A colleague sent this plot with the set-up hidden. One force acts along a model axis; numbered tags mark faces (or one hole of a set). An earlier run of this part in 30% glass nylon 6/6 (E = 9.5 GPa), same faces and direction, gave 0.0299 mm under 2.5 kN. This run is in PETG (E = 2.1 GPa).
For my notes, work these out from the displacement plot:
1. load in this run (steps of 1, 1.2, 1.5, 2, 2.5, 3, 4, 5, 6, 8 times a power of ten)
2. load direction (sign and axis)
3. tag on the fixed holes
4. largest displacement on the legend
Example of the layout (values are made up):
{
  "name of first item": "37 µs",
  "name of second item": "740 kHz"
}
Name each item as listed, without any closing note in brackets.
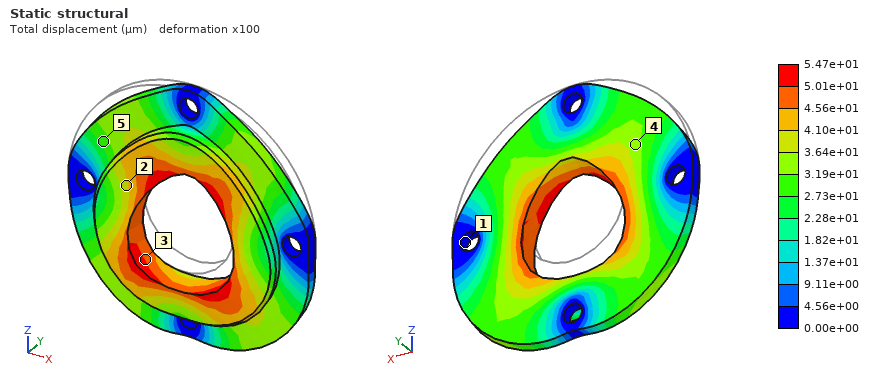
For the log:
{
  "load in this run": "1 kN",
  "load direction": "-Z",
  "tag on the fixed holes": "1",
  "largest displacement on the legend": "5.47e+01 µm"
}
